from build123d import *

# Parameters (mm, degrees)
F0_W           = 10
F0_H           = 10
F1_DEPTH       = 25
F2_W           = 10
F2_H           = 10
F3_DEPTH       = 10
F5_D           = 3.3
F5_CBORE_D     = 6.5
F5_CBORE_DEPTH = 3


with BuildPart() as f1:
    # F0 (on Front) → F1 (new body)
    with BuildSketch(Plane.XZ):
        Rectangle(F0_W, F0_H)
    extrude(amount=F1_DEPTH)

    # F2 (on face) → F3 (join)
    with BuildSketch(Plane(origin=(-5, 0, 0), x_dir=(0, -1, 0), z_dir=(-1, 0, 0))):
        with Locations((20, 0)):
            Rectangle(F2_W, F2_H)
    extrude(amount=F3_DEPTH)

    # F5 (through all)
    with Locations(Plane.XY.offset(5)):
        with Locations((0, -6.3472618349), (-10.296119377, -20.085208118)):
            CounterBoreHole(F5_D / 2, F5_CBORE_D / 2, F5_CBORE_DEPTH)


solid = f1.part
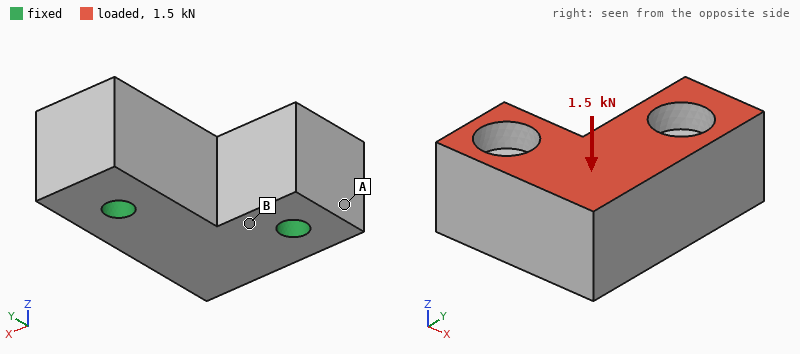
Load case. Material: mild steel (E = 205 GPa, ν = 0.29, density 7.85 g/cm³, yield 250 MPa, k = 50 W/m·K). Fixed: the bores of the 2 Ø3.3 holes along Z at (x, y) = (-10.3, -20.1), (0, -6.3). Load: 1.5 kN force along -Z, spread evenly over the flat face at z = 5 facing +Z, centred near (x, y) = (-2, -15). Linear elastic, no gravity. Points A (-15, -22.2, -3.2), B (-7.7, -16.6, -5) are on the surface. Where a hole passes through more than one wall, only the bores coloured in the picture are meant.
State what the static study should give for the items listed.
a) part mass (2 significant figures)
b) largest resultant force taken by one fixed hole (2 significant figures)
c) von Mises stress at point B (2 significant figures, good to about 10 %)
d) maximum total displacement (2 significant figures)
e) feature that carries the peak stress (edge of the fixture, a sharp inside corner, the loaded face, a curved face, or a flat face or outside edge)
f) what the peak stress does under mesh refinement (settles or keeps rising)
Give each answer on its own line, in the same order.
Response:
25 g
770 N
13 MPa
3.6 µm
edge of the fixture
keeps rising
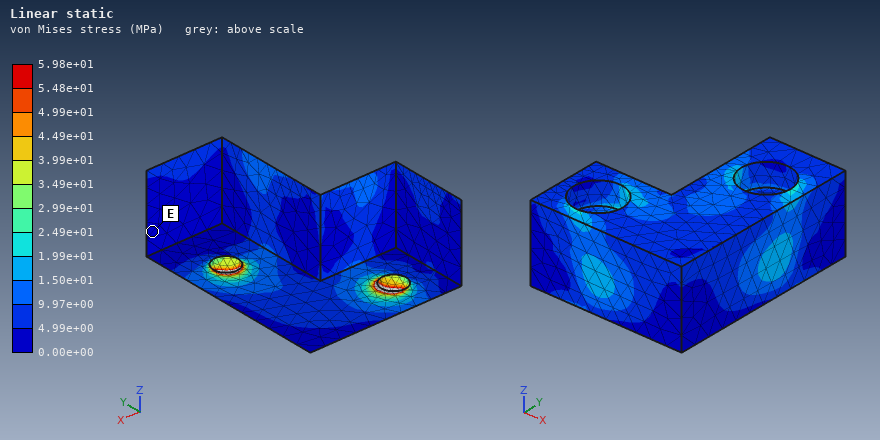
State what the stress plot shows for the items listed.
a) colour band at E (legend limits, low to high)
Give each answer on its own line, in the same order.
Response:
0.00e+00 to 4.99e+00 MPa
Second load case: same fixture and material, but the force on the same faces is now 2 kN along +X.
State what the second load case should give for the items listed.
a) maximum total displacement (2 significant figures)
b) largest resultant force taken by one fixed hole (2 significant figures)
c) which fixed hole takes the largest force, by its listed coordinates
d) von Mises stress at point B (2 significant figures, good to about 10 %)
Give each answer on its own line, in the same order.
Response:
5.4 µm
1.3 kN
(-10.3, -20.1)
14 MPa
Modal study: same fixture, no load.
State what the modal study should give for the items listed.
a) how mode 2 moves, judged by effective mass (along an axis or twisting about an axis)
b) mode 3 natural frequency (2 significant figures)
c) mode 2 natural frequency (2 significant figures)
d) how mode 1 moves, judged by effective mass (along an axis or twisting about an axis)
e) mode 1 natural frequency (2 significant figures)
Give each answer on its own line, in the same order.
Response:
along Y
64 kHz
59 kHz
along Z
29 kHz
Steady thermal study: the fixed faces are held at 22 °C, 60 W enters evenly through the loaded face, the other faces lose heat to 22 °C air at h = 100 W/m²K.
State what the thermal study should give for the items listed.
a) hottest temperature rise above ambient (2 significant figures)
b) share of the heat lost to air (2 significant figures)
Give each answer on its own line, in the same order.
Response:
56 K
4.8 %
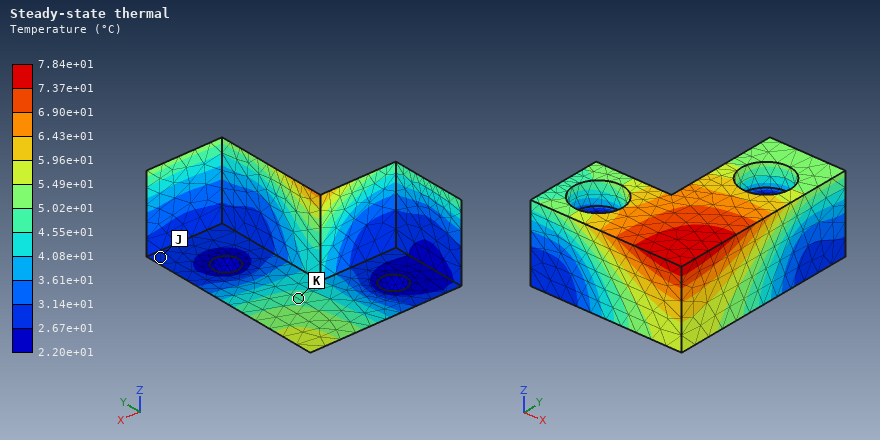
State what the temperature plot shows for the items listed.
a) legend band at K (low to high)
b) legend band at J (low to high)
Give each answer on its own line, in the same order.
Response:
4.55e+01 to 5.02e+01 °C
2.67e+01 to 3.14e+01 °C
